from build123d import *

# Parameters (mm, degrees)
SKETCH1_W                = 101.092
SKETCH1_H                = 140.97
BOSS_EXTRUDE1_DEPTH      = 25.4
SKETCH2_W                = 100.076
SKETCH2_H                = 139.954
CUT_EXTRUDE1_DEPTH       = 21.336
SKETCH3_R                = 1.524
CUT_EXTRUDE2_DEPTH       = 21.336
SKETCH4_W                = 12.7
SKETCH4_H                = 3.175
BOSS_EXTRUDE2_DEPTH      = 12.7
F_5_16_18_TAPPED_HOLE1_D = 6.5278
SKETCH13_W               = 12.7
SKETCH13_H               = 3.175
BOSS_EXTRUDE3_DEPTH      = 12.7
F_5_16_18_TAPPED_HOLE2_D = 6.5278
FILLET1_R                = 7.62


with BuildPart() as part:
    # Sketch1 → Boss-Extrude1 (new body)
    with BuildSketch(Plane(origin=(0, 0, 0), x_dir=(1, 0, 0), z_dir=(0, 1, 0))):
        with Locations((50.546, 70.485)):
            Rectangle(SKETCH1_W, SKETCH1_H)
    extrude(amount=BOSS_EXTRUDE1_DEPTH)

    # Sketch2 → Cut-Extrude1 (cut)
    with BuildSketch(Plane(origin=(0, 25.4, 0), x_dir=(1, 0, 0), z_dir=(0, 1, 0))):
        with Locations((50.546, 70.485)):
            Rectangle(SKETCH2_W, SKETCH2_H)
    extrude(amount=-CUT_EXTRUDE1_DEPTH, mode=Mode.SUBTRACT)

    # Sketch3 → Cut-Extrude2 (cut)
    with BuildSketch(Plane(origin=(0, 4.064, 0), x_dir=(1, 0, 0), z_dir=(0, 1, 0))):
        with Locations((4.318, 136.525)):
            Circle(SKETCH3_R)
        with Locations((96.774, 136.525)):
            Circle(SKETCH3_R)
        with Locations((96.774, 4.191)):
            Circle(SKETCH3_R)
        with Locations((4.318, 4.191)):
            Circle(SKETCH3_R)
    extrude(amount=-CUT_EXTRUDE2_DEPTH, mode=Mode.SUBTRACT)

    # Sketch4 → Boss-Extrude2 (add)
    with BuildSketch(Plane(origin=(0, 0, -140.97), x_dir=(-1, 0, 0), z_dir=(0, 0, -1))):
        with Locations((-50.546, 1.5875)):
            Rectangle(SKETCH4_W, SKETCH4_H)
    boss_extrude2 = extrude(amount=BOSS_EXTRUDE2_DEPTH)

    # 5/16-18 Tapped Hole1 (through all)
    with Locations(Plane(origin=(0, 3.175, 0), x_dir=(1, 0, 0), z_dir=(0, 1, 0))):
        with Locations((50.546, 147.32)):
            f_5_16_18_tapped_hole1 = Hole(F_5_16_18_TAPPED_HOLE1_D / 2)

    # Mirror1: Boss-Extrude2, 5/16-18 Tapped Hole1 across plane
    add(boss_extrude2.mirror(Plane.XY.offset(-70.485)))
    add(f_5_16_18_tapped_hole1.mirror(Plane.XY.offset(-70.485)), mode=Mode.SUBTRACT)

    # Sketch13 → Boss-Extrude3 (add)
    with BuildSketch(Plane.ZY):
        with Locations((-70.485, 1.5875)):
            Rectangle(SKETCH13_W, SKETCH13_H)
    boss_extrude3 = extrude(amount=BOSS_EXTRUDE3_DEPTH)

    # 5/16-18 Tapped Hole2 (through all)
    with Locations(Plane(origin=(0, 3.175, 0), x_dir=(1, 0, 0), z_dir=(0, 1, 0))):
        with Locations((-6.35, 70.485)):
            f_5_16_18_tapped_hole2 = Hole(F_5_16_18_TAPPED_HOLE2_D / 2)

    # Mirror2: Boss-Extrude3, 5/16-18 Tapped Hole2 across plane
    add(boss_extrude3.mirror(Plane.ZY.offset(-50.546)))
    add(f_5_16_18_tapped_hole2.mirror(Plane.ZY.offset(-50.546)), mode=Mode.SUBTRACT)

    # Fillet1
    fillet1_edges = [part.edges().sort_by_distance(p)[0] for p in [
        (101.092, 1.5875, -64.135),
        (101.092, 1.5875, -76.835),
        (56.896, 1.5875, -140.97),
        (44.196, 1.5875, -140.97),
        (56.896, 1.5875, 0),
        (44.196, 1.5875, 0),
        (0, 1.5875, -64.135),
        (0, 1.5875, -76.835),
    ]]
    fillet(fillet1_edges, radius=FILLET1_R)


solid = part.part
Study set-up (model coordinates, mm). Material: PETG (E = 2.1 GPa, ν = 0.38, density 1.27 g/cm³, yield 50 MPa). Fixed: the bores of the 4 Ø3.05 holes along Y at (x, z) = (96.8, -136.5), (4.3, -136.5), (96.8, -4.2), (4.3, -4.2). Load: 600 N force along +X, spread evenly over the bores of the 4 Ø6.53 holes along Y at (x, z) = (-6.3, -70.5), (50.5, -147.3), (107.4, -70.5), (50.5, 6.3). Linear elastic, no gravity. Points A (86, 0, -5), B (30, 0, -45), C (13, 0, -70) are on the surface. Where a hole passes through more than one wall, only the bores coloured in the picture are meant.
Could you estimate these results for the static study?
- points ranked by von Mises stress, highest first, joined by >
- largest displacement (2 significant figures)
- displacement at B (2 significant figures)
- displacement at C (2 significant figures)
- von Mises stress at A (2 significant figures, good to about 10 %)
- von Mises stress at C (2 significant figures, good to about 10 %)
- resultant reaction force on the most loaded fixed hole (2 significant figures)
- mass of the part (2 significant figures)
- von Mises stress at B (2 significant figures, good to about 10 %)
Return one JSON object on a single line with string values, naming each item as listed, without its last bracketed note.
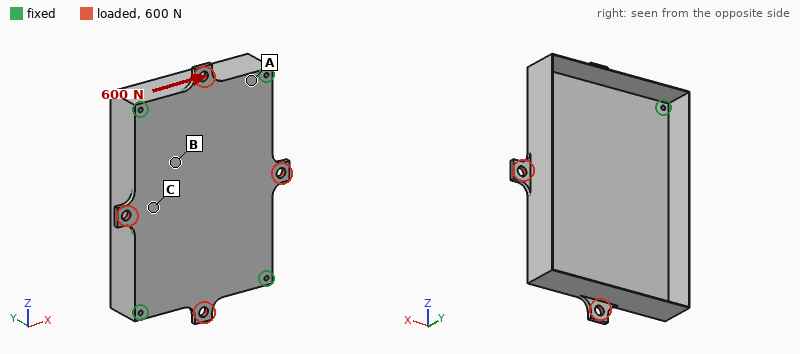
{"points ranked by von Mises stress, highest first, joined by >": "A > C > B", "largest displacement": "0.16 mm", "displacement at B": "0.048 mm", "displacement at C": "0.064 mm", "von Mises stress at A": "2.7 MPa", "von Mises stress at C": "1.4 MPa", "resultant reaction force on the most loaded fixed hole": "160 N", "mass of the part": "83 g", "von Mises stress at B": "0.86 MPa"}
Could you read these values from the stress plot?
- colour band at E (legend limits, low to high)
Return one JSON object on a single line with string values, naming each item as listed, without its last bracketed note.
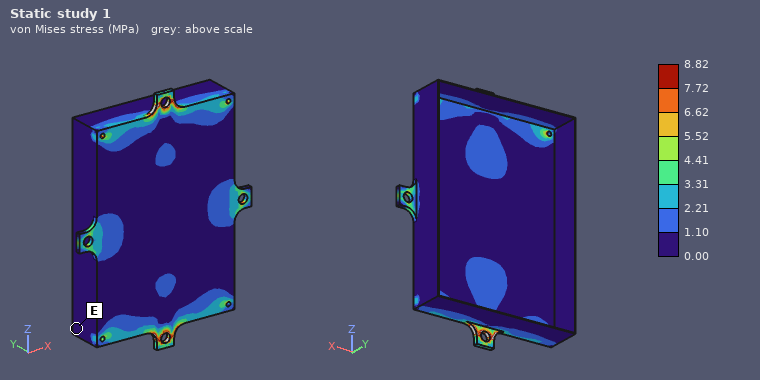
{"colour band at E": "0.00 to 1.10 MPa"}
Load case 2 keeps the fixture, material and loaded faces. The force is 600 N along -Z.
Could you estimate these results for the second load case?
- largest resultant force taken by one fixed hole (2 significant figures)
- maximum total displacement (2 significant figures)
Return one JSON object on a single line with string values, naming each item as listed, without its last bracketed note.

{"largest resultant force taken by one fixed hole": "160 N", "maximum total displacement": "0.17 mm"}
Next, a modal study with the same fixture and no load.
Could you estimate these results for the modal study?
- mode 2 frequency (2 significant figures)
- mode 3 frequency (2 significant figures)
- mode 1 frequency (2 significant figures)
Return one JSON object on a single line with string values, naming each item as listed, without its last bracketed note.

{"mode 2 frequency": "310 Hz", "mode 3 frequency": "310 Hz", "mode 1 frequency": "300 Hz"}
